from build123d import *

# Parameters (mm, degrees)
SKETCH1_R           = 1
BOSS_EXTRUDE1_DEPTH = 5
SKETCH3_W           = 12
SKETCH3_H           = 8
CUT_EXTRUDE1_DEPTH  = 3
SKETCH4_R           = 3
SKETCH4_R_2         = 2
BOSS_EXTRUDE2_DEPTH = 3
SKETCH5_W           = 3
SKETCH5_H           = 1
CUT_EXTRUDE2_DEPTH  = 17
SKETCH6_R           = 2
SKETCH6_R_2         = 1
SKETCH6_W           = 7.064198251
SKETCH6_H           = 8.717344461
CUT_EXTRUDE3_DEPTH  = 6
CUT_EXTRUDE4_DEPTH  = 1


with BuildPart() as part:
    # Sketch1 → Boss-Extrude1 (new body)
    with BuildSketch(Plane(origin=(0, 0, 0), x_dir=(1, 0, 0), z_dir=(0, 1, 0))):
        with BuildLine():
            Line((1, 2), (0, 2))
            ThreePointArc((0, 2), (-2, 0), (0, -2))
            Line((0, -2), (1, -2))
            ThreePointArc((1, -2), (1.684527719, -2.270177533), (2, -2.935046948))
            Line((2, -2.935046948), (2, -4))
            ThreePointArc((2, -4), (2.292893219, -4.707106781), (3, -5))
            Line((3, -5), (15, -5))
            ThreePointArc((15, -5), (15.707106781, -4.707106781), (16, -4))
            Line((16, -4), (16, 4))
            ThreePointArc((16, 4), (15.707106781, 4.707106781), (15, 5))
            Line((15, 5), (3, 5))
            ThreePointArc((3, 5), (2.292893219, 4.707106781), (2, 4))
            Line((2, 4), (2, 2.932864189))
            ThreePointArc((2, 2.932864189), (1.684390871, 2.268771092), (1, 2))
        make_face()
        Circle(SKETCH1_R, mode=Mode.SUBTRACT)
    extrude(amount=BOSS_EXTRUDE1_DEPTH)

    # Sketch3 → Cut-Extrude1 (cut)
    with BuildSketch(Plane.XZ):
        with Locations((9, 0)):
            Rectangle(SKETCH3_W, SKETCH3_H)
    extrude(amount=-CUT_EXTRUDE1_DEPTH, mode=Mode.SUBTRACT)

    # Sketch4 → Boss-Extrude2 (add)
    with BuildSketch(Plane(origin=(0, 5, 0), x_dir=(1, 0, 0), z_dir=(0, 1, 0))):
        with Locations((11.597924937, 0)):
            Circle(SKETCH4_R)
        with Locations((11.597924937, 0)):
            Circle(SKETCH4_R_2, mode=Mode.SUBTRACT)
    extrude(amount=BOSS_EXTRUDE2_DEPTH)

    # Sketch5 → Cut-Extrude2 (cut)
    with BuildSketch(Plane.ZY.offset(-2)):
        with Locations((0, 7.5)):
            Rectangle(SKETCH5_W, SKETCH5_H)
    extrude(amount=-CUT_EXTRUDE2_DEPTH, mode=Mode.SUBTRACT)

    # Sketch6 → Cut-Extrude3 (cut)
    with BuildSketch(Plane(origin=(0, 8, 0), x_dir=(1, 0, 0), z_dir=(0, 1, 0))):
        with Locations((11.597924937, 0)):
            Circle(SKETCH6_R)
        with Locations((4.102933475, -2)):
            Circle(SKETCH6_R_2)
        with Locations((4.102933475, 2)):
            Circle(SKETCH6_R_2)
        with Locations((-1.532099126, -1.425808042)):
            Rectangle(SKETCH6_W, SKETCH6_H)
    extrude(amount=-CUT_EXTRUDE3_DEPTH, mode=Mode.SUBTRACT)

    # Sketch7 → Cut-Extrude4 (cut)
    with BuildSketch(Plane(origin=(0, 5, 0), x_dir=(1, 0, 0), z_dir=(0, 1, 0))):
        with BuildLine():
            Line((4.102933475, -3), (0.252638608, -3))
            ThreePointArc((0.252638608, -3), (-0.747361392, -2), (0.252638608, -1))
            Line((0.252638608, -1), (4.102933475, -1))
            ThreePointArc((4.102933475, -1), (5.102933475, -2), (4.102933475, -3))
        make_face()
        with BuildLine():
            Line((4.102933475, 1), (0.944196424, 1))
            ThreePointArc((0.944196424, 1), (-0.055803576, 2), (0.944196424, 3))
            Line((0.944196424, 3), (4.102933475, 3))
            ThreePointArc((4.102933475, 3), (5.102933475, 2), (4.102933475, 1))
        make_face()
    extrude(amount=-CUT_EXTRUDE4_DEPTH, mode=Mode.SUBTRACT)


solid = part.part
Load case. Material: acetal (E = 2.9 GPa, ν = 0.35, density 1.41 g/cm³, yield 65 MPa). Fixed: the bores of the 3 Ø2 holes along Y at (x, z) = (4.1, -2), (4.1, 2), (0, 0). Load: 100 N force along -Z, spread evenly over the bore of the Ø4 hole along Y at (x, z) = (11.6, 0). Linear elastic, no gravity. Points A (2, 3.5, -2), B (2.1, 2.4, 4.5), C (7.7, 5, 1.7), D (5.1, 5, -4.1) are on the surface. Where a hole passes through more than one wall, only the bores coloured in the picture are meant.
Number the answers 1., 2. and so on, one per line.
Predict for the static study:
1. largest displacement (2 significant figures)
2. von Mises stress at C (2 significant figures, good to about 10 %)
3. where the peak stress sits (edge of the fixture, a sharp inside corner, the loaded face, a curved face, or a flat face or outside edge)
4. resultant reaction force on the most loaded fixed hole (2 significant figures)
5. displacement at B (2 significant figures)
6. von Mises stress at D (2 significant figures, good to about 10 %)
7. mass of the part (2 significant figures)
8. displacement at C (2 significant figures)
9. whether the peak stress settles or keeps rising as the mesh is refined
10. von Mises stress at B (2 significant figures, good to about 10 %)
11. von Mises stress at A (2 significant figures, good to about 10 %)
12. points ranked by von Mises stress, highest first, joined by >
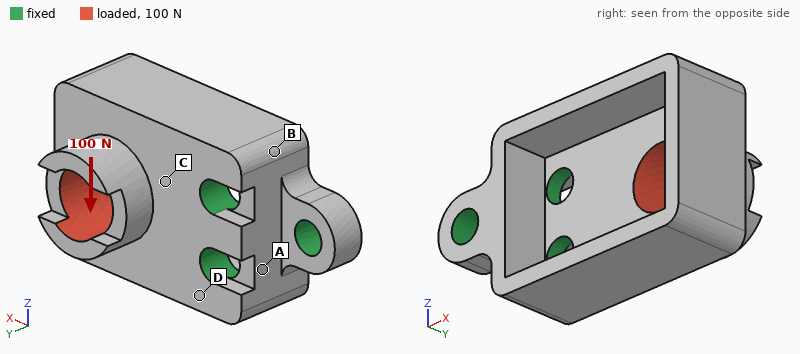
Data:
1. 0.18 mm
2. 18 MPa
3. edge of the fixture
4. 120 N
5. 0.031 mm
6. 7.1 MPa
7. 0.60 g
8. 0.038 mm
9. keeps rising
10. 3.4 MPa
11. 13 MPa
12. C > A > D > B
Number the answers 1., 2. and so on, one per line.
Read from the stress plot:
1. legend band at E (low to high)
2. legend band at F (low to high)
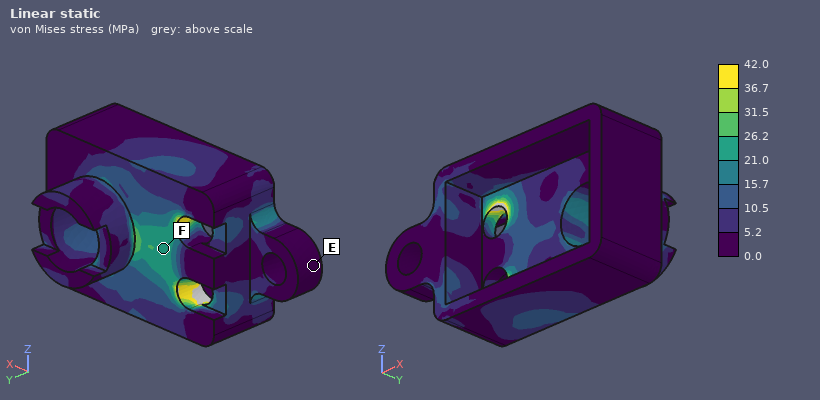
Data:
1. 0.0 to 5.2 MPa
2. 21.0 to 26.2 MPa
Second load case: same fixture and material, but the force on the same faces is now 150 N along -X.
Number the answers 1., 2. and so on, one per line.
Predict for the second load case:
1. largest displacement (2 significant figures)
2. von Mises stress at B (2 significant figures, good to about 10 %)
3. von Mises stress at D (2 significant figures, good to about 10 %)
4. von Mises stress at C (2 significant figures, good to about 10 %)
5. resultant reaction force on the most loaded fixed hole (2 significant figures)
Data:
1. 0.23 mm
2. 6.1 MPa
3. 12 MPa
4. 22 MPa
5. 80 N
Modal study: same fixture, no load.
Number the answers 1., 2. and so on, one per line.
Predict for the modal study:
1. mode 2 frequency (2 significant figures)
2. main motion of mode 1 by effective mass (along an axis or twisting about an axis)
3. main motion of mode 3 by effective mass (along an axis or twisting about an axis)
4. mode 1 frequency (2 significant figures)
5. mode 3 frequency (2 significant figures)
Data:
1. 5800 Hz
2. along Y
3. along Z
4. 3900 Hz
5. 7900 Hz
